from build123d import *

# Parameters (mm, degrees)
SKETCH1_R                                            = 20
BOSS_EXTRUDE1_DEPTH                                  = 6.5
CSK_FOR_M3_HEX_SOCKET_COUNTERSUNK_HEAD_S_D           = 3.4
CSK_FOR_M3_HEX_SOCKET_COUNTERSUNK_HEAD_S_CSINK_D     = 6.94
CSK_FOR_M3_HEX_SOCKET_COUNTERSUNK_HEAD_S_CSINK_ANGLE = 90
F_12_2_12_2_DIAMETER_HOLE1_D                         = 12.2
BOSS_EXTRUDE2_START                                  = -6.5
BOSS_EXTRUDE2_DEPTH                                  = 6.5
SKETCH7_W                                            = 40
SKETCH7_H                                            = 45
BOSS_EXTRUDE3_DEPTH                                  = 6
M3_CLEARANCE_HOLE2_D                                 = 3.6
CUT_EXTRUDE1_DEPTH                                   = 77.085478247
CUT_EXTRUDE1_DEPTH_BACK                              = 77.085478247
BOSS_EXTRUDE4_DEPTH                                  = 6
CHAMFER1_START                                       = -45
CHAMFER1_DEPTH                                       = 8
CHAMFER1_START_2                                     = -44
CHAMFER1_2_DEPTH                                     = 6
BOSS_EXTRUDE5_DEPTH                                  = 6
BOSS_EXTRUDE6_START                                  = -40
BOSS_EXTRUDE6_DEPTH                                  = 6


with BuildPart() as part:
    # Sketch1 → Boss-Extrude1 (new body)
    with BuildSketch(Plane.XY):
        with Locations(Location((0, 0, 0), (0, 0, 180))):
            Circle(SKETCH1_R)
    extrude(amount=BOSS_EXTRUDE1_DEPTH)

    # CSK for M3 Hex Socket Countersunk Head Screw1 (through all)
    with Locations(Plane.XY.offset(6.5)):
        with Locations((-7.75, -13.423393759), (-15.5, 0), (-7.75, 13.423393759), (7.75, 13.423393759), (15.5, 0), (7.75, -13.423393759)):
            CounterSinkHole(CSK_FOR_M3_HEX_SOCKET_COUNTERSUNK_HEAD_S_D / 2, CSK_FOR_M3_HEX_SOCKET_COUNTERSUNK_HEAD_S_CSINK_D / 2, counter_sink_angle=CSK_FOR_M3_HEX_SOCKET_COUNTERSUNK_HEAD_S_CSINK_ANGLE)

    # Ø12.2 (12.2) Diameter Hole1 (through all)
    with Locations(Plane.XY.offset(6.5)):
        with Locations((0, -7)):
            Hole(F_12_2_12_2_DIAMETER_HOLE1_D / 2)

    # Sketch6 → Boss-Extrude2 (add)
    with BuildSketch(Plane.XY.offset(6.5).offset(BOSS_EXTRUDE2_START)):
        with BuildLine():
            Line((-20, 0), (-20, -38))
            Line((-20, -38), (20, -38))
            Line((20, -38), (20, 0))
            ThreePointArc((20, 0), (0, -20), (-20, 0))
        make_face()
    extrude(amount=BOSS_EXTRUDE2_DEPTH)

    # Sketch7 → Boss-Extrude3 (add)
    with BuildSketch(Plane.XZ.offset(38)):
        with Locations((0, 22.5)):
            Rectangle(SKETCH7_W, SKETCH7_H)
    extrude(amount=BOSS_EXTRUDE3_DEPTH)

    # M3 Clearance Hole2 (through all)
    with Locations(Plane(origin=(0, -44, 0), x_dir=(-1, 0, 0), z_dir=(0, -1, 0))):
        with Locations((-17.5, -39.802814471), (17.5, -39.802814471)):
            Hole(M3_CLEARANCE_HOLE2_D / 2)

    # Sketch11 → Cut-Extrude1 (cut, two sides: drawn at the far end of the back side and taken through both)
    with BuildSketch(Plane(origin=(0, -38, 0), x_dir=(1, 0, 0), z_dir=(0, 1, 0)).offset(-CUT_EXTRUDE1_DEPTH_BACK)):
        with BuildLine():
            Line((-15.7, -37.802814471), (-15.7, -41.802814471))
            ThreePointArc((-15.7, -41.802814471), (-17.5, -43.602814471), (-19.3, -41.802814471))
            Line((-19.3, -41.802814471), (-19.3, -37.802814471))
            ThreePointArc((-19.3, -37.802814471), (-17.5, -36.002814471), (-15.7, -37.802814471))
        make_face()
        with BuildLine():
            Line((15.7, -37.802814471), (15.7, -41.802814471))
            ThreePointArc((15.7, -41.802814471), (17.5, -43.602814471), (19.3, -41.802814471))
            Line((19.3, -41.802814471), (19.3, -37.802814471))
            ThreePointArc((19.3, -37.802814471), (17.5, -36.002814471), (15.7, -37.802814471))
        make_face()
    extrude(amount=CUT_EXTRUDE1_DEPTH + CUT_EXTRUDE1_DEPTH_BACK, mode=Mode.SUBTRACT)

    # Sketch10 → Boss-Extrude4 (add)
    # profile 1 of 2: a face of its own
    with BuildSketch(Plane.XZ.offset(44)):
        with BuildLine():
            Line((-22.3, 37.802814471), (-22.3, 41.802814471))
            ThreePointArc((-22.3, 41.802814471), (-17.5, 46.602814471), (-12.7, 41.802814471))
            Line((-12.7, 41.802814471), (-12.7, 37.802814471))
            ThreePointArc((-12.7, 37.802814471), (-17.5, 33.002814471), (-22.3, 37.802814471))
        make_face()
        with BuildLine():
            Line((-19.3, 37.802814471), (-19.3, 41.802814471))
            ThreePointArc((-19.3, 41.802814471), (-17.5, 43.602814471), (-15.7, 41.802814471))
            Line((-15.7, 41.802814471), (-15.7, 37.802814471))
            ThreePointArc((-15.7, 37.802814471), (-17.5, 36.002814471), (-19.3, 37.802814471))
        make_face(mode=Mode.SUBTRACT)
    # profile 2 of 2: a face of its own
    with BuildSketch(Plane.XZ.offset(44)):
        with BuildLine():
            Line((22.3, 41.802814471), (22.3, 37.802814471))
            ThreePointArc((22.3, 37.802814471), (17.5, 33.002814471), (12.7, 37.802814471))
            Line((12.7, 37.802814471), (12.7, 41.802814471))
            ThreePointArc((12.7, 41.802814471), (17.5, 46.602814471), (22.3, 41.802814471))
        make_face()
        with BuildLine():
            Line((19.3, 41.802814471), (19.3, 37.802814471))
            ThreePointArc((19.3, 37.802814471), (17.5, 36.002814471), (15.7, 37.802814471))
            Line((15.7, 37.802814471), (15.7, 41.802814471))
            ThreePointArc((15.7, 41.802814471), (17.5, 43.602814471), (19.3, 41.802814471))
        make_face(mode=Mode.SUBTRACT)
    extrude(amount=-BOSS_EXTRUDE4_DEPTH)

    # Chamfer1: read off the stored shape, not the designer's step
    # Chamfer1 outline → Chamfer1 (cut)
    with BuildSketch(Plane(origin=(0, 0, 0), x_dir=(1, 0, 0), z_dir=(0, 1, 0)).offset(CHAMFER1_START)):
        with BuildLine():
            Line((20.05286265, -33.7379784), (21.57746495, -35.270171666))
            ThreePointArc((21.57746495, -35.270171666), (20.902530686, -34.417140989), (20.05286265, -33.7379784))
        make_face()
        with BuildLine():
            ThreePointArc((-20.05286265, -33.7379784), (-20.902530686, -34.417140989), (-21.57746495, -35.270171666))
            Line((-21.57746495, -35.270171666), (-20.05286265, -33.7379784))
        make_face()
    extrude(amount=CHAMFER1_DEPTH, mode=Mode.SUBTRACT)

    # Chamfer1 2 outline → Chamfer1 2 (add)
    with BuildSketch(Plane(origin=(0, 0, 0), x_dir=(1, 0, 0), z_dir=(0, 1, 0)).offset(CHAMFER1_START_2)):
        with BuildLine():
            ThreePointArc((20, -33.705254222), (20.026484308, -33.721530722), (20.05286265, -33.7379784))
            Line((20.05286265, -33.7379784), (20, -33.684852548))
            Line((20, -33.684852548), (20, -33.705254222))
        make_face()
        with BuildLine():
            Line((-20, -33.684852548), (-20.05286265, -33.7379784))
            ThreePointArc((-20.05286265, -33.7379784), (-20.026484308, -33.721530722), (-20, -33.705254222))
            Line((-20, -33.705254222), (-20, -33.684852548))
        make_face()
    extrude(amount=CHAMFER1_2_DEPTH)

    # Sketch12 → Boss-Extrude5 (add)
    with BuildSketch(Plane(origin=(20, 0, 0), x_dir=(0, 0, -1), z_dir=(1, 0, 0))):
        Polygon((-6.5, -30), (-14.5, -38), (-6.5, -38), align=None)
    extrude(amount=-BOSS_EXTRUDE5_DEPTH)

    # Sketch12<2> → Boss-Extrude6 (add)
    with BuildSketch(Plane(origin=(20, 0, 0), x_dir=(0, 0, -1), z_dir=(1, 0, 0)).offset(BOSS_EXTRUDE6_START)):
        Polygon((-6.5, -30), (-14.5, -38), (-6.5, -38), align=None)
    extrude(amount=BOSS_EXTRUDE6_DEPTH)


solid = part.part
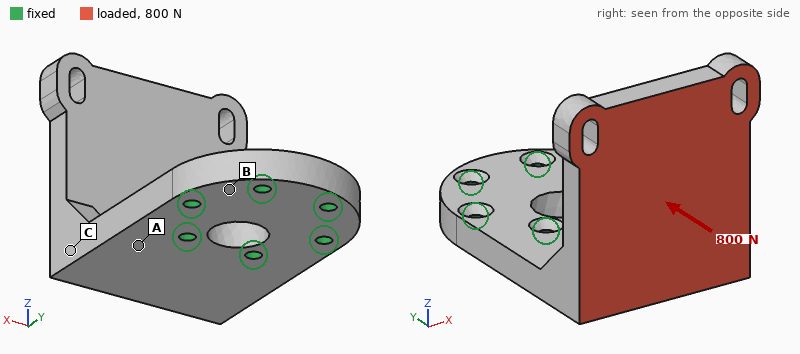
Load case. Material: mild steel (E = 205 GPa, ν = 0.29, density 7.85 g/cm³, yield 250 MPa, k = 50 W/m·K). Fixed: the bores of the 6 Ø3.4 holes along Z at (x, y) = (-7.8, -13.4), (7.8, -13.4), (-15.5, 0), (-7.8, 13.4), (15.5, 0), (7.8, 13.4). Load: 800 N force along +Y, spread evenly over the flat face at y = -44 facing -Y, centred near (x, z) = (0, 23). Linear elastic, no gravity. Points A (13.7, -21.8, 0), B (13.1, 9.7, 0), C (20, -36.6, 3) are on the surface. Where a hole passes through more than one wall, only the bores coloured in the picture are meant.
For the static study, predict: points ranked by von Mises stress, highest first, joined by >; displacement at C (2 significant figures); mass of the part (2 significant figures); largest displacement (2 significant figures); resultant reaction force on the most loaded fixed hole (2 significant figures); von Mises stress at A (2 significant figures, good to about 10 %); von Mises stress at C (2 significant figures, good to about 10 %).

A > C > B
0.027 mm
190 g
0.13 mm
350 N
51 MPa
29 MPa
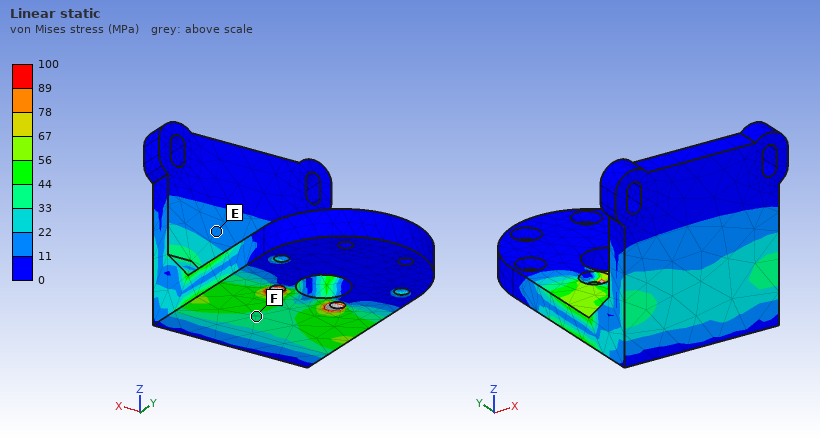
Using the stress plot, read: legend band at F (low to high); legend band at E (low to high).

33 to 44 MPa
11 to 22 MPa
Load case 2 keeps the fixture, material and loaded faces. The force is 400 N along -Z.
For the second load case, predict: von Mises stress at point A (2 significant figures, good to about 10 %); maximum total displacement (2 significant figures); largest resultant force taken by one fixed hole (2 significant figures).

30 MPa
58 µm
390 N
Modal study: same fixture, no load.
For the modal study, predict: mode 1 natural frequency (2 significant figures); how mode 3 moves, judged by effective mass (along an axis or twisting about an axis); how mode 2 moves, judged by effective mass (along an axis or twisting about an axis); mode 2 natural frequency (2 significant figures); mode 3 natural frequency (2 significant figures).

1500 Hz
along Z
along X
2500 Hz
4300 Hz
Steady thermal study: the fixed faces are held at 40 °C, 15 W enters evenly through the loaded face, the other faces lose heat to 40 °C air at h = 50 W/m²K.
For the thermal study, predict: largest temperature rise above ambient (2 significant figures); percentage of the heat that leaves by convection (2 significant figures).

35 K
37 %
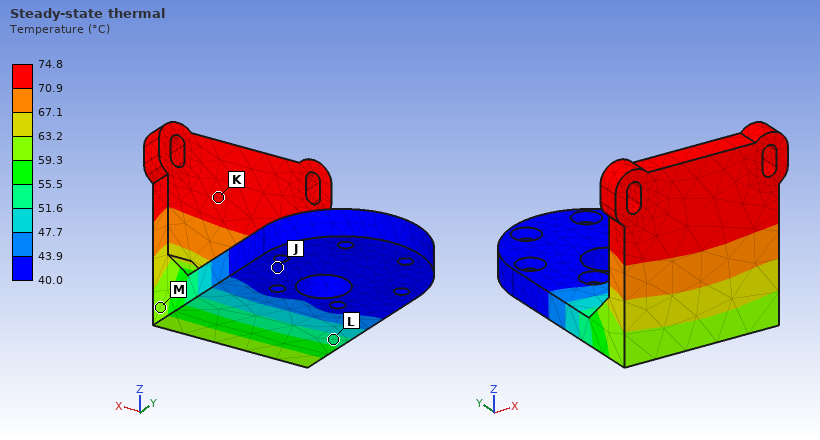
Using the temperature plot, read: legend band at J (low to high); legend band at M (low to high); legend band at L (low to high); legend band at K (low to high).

40.0 to 43.9 °C
59.3 to 63.2 °C
51.6 to 55.5 °C
70.9 to 74.8 °C
